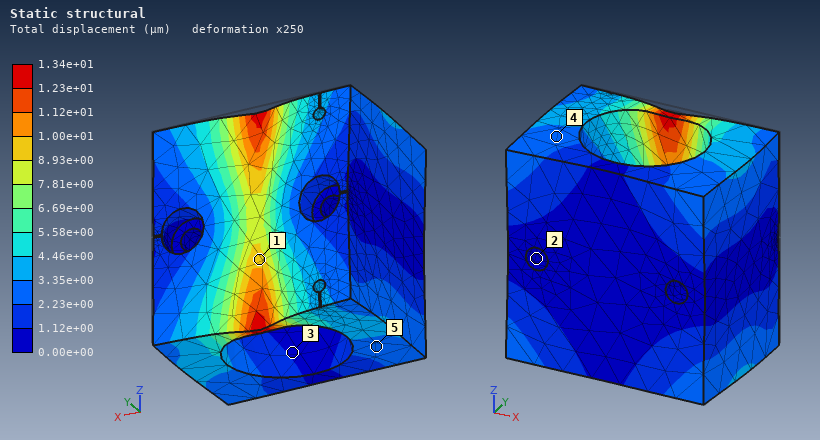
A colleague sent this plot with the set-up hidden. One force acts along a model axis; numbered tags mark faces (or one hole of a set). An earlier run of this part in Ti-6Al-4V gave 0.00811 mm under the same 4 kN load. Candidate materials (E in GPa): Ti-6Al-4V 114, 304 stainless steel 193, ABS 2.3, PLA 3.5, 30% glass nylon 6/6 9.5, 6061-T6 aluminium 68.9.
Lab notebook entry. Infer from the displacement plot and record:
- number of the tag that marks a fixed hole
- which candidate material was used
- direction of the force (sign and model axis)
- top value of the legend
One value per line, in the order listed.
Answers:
2
6061-T6 aluminium
-Y
1.34e+01 µm
